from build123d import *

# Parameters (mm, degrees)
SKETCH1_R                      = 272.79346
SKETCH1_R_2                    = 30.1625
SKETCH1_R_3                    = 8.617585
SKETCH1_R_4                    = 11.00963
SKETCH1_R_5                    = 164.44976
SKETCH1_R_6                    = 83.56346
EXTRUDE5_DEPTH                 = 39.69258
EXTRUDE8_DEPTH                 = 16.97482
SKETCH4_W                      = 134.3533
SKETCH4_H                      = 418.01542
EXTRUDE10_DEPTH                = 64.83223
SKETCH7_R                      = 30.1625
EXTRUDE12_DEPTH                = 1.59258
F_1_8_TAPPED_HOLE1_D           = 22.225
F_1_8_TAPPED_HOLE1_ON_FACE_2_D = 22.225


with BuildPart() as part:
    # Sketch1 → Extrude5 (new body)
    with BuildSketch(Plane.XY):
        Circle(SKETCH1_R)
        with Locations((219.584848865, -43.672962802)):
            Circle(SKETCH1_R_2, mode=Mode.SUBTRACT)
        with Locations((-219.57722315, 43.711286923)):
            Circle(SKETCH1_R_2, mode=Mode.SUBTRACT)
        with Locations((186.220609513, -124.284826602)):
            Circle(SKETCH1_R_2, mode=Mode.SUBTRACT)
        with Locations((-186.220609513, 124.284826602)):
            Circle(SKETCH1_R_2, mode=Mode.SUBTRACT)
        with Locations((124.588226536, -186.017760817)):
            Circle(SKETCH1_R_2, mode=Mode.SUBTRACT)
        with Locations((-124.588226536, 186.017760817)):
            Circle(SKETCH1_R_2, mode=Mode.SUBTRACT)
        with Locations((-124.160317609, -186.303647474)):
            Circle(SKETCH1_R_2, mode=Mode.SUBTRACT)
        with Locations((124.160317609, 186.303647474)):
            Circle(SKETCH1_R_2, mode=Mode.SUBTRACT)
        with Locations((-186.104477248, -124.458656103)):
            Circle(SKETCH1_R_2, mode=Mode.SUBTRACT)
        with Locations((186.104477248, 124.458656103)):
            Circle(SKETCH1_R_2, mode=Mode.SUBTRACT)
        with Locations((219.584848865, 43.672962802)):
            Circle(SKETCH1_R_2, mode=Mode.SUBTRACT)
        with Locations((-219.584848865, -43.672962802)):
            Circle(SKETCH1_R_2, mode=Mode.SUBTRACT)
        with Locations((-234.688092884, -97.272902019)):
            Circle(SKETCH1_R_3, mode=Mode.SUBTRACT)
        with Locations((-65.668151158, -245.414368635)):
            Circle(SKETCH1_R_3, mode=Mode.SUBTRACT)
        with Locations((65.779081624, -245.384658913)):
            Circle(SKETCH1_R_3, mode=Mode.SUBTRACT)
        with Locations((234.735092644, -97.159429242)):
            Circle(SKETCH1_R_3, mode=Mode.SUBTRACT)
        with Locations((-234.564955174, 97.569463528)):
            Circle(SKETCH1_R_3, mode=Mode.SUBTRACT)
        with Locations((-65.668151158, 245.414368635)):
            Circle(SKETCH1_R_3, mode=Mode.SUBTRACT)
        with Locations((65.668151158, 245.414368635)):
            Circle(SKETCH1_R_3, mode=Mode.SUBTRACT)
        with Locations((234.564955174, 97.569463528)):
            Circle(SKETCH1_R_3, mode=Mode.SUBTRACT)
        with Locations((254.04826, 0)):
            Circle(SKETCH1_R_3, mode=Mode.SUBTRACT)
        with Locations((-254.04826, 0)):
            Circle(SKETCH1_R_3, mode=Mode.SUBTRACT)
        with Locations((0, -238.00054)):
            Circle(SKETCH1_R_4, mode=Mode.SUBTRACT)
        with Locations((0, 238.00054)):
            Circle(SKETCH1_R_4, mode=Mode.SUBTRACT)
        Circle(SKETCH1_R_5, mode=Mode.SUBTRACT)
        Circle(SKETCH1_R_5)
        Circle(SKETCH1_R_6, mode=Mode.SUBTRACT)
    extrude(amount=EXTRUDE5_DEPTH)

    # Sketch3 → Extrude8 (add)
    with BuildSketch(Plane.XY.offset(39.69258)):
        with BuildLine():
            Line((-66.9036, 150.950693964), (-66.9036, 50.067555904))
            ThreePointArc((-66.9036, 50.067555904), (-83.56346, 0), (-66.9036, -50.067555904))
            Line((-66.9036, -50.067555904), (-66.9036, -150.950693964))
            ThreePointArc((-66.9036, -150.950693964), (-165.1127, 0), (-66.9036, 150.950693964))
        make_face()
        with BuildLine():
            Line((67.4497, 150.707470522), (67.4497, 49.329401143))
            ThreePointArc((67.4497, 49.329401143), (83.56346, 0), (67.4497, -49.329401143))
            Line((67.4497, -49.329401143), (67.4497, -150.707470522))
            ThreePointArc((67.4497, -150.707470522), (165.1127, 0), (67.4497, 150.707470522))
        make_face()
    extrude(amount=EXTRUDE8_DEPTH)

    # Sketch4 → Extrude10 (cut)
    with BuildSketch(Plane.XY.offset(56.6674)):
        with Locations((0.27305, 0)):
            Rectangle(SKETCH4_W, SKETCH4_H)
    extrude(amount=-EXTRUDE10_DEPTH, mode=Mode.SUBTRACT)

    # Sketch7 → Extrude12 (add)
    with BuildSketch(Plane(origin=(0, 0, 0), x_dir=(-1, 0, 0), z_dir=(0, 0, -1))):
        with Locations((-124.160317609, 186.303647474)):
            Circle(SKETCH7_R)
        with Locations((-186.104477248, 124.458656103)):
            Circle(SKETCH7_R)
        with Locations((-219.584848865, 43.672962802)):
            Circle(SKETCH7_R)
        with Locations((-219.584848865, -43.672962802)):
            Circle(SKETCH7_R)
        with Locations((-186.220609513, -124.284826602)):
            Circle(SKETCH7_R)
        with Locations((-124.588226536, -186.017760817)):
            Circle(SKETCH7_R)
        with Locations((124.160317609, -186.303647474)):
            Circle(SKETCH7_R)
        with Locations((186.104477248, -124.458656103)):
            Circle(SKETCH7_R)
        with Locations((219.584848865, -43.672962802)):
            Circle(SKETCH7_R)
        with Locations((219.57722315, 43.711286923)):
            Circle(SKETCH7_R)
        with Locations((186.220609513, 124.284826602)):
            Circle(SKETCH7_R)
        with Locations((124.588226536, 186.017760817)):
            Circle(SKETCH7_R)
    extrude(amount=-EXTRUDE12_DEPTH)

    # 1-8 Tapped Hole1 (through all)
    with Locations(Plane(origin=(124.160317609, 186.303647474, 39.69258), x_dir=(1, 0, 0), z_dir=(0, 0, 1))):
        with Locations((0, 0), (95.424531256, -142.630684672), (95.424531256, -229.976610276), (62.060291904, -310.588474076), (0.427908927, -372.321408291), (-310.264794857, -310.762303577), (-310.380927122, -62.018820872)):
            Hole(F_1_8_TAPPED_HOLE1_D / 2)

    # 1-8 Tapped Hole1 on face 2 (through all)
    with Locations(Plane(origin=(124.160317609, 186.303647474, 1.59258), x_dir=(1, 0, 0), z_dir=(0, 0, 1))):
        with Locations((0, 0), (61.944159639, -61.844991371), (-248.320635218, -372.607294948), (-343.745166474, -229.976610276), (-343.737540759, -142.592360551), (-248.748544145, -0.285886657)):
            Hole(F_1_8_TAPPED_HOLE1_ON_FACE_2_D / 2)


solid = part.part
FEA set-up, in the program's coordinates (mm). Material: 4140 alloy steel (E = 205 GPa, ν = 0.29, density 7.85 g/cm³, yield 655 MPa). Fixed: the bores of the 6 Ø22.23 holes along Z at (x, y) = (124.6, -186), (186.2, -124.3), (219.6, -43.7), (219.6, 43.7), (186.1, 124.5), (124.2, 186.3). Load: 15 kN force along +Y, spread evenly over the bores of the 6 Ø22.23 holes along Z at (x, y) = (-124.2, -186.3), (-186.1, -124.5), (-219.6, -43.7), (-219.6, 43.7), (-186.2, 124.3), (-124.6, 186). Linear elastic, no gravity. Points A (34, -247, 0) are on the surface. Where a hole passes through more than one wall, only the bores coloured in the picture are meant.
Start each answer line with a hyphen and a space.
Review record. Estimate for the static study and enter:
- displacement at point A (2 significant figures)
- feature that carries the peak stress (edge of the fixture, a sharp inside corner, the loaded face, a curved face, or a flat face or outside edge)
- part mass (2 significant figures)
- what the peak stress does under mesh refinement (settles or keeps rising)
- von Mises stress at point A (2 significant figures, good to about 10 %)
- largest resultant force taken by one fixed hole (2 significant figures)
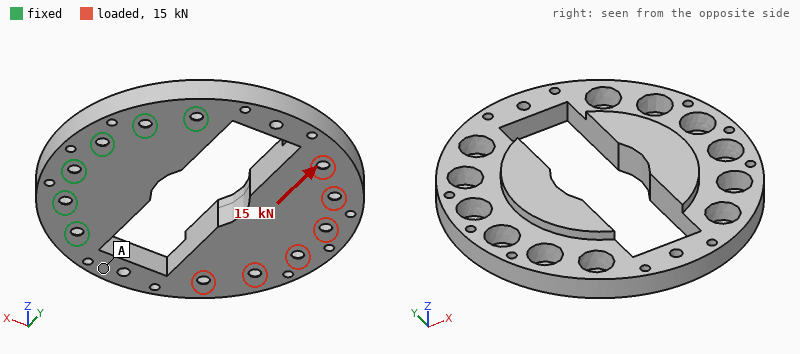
- 0.060 mm
- edge of the fixture
- 49 kg
- keeps rising
- 12 MPa
- 11 kN
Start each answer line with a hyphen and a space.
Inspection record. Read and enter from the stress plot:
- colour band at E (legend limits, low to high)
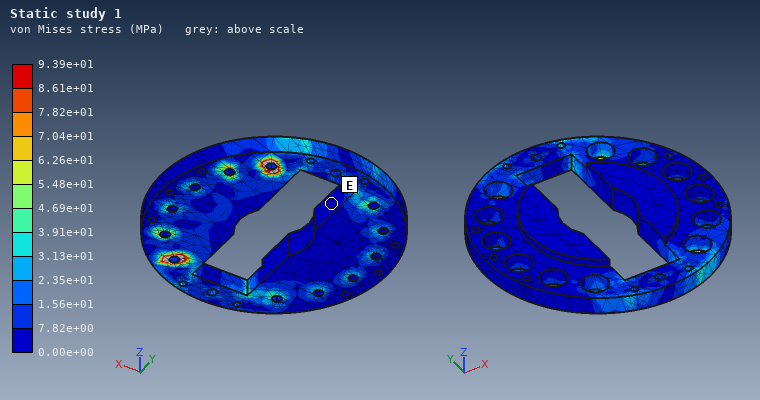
- 0.00e+00 to 7.82e+00 MPa
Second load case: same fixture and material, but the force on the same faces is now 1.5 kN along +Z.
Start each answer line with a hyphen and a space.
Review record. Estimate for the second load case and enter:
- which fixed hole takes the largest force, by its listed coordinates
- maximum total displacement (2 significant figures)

- (124.2, 186.3)
- 0.65 mm
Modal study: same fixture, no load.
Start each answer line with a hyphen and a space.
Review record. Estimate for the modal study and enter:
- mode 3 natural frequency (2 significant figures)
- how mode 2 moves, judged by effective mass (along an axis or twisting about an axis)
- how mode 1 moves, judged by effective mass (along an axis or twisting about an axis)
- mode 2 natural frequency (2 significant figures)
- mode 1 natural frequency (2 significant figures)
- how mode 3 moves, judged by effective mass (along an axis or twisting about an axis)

- 360 Hz
- twisting about X
- along Z
- 290 Hz
- 64 Hz
- along Y
